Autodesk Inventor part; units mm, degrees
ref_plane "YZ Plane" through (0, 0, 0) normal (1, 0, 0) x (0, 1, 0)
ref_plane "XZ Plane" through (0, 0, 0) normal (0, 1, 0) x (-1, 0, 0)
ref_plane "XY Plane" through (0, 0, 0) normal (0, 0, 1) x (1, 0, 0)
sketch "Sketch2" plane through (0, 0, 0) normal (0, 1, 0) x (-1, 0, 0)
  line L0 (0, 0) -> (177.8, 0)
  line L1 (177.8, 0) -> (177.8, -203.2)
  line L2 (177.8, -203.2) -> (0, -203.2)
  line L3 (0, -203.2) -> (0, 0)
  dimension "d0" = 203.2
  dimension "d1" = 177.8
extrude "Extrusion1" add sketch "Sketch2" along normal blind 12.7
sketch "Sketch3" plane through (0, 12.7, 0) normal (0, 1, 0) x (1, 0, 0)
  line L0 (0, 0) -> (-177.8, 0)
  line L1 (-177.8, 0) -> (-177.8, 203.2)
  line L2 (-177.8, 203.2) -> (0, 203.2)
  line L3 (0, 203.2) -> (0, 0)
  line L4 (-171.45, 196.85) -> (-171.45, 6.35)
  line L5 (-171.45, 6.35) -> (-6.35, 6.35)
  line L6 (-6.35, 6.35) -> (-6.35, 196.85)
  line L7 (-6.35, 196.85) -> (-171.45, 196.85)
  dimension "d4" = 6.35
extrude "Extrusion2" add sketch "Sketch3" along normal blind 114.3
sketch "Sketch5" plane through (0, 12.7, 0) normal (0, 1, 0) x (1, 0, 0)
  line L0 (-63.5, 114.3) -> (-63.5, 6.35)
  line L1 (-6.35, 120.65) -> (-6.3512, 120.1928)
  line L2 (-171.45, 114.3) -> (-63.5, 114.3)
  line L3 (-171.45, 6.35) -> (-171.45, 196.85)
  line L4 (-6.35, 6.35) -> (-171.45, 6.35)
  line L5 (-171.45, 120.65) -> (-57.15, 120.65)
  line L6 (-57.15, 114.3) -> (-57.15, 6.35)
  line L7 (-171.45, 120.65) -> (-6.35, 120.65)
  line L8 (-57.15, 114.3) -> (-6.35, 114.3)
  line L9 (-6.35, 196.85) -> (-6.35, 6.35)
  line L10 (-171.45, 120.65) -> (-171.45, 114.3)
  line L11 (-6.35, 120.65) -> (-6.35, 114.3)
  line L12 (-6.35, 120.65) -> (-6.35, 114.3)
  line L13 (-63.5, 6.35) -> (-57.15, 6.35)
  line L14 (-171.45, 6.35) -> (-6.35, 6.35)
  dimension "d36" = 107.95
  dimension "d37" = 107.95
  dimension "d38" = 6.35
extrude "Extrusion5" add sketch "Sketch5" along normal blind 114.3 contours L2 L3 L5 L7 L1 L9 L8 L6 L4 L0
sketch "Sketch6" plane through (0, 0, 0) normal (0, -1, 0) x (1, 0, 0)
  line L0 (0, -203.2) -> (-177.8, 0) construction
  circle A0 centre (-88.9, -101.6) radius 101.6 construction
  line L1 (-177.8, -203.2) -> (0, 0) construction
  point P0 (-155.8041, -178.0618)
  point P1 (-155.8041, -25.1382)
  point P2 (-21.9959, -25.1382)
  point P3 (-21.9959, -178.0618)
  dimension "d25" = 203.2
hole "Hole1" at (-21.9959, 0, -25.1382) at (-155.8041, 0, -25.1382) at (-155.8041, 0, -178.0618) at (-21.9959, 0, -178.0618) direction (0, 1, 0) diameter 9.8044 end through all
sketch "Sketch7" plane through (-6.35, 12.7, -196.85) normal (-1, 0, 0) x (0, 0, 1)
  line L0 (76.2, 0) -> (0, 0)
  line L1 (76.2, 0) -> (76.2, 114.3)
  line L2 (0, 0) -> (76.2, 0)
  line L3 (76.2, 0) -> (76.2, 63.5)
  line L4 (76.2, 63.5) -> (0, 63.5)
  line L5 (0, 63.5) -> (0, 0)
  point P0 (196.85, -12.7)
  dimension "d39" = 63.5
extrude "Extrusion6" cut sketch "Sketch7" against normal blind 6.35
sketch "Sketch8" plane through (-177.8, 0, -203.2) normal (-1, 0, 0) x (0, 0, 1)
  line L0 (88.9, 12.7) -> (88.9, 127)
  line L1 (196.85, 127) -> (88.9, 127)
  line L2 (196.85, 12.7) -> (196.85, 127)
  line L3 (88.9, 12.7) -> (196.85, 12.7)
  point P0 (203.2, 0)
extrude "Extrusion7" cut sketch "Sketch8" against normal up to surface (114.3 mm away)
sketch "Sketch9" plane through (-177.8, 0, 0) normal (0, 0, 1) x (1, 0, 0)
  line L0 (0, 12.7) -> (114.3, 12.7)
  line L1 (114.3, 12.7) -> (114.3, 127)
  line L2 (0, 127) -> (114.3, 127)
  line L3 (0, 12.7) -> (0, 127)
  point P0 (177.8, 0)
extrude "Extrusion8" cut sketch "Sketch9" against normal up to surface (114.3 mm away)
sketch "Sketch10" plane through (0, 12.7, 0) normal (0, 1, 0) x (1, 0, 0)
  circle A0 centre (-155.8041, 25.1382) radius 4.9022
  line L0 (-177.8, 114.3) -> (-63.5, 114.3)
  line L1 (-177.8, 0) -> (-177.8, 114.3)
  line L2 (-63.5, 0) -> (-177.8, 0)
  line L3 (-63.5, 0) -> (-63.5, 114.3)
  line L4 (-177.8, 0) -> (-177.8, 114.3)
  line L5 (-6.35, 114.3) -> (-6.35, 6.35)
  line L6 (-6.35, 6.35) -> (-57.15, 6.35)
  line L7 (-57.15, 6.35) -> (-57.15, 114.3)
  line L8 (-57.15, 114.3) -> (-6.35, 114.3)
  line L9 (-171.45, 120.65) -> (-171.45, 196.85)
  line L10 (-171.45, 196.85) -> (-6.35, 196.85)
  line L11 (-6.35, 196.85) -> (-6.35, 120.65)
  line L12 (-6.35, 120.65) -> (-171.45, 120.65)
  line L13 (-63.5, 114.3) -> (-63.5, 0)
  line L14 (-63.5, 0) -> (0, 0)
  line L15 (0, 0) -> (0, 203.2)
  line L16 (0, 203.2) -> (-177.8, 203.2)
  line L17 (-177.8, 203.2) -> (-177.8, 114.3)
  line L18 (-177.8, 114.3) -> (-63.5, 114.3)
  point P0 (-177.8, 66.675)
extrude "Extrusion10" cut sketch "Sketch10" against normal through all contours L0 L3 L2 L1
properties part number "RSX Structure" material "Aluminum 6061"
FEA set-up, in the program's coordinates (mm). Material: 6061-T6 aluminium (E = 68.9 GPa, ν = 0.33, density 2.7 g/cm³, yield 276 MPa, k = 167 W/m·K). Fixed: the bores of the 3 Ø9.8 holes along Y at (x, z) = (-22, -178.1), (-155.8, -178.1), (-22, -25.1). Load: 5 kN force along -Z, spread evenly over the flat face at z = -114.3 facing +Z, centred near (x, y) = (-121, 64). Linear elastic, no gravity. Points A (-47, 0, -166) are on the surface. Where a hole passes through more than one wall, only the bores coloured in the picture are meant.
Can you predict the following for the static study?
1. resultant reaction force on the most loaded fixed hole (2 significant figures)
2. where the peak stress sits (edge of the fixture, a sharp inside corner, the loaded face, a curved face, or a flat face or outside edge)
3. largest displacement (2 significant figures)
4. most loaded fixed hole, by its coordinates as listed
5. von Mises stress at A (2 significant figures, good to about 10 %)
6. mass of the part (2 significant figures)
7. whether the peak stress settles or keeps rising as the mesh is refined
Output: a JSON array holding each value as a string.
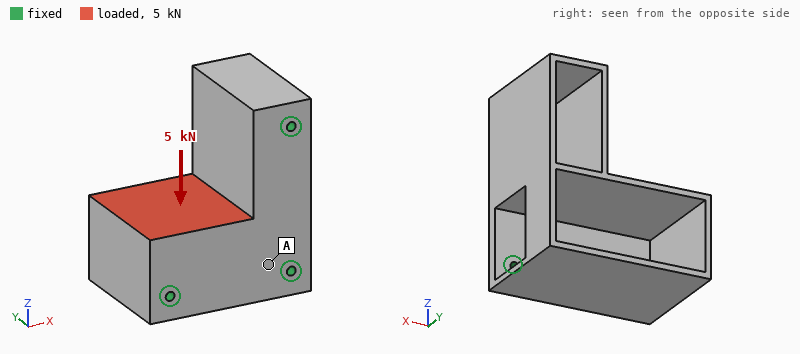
["2.8 kN", "edge of the fixture", "0.35 mm", "(-155.8, -178.1)", "4.2 MPa", "2.2 kg", "keeps rising"]
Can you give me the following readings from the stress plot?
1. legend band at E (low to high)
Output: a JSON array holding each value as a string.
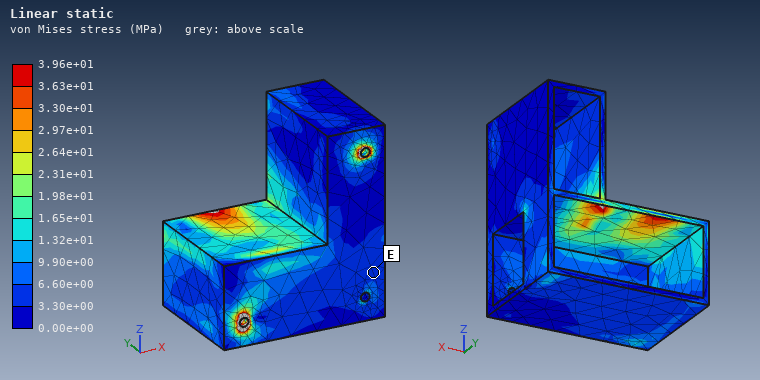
["3.30e+00 to 6.60e+00 MPa"]
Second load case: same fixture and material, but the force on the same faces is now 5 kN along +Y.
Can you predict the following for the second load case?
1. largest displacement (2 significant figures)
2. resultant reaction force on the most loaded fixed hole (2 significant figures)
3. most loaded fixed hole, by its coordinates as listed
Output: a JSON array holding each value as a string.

["0.31 mm", "3.2 kN", "(-155.8, -178.1)"]
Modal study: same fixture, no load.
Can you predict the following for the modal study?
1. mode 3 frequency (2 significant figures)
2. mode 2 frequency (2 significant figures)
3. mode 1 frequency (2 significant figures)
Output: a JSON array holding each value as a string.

["1300 Hz", "1100 Hz", "790 Hz"]
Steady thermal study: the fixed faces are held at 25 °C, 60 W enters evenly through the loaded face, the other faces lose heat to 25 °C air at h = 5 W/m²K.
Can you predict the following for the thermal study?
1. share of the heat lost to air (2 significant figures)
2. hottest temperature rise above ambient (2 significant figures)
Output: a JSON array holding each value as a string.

["9.3 %", "17 K"]
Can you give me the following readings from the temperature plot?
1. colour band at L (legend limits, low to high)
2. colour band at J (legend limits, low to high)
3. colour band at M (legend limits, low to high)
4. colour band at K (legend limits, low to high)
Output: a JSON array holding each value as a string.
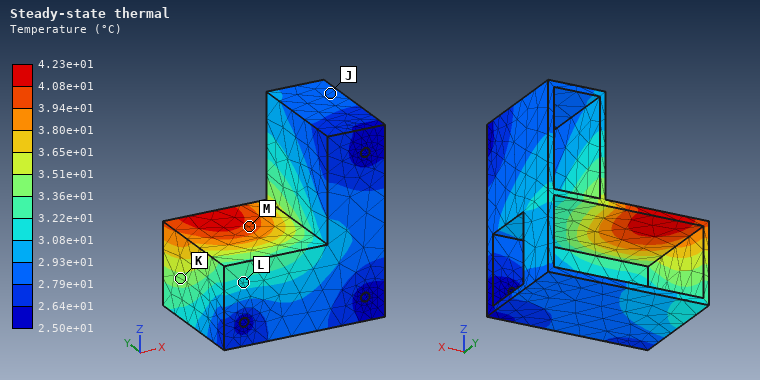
["3.08e+01 to 3.22e+01 °C", "2.79e+01 to 2.93e+01 °C", "3.94e+01 to 4.08e+01 °C", "3.36e+01 to 3.51e+01 °C"]
